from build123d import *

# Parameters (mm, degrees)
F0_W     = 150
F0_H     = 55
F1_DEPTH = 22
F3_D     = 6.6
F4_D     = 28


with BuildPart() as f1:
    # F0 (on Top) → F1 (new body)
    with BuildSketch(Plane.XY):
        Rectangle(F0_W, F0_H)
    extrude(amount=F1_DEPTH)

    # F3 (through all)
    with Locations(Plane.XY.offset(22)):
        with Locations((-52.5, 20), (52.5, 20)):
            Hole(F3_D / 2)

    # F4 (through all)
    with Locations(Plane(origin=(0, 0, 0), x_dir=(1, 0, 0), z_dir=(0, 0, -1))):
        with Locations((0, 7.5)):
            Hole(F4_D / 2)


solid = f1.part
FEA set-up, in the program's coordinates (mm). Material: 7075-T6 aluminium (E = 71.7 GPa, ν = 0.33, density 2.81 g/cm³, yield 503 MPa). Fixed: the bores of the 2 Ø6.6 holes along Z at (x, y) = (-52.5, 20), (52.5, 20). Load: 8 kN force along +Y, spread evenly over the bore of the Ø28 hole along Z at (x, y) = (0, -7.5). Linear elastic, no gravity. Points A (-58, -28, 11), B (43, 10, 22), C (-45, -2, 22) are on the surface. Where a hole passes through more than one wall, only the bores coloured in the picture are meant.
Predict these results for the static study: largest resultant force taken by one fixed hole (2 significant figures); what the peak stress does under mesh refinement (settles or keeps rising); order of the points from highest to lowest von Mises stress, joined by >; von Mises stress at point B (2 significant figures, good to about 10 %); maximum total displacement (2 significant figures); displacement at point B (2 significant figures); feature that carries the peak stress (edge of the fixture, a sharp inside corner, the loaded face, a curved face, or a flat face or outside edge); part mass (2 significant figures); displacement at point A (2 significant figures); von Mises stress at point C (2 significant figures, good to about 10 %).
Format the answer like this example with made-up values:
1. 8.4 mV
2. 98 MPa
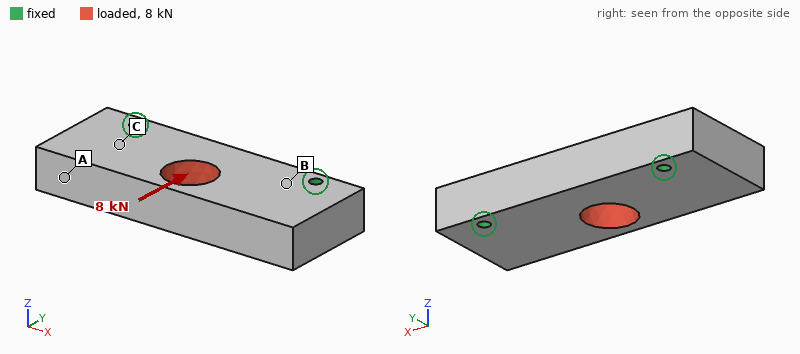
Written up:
1. 4.8 kN
2. keeps rising
3. B > C > A
4. 10 MPa
5. 15 µm
6. 3.5 µm
7. edge of the fixture
8. 470 g
9. 7.0 µm
10. 6.3 MPa
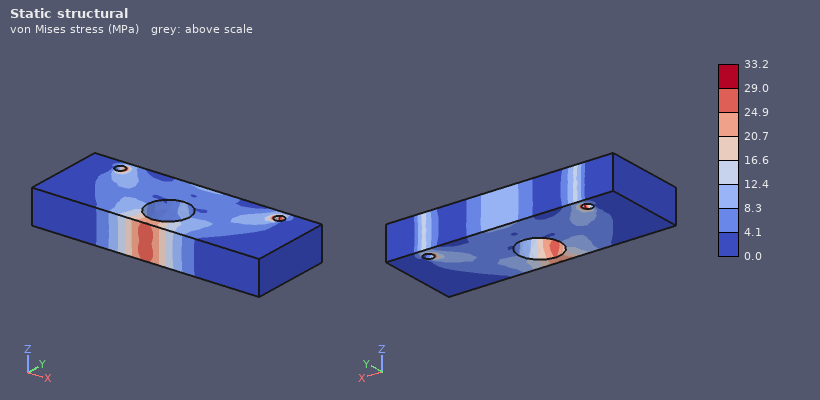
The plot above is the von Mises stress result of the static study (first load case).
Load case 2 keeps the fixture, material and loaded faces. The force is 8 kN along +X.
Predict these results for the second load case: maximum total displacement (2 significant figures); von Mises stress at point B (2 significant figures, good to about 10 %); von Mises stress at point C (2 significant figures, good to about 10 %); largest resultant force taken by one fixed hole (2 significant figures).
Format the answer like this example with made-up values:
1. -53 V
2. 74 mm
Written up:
1. 10 µm
2. 6.6 MPa
3. 3.5 MPa
4. 4.4 kN
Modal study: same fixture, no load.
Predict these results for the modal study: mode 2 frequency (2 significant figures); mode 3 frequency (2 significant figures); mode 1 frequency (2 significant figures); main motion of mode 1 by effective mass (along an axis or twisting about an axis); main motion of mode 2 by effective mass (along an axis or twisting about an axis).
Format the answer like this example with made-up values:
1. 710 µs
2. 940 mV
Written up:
1. 6300 Hz
2. 7300 Hz
3. 4200 Hz
4. along Z
5. twisting about Y
